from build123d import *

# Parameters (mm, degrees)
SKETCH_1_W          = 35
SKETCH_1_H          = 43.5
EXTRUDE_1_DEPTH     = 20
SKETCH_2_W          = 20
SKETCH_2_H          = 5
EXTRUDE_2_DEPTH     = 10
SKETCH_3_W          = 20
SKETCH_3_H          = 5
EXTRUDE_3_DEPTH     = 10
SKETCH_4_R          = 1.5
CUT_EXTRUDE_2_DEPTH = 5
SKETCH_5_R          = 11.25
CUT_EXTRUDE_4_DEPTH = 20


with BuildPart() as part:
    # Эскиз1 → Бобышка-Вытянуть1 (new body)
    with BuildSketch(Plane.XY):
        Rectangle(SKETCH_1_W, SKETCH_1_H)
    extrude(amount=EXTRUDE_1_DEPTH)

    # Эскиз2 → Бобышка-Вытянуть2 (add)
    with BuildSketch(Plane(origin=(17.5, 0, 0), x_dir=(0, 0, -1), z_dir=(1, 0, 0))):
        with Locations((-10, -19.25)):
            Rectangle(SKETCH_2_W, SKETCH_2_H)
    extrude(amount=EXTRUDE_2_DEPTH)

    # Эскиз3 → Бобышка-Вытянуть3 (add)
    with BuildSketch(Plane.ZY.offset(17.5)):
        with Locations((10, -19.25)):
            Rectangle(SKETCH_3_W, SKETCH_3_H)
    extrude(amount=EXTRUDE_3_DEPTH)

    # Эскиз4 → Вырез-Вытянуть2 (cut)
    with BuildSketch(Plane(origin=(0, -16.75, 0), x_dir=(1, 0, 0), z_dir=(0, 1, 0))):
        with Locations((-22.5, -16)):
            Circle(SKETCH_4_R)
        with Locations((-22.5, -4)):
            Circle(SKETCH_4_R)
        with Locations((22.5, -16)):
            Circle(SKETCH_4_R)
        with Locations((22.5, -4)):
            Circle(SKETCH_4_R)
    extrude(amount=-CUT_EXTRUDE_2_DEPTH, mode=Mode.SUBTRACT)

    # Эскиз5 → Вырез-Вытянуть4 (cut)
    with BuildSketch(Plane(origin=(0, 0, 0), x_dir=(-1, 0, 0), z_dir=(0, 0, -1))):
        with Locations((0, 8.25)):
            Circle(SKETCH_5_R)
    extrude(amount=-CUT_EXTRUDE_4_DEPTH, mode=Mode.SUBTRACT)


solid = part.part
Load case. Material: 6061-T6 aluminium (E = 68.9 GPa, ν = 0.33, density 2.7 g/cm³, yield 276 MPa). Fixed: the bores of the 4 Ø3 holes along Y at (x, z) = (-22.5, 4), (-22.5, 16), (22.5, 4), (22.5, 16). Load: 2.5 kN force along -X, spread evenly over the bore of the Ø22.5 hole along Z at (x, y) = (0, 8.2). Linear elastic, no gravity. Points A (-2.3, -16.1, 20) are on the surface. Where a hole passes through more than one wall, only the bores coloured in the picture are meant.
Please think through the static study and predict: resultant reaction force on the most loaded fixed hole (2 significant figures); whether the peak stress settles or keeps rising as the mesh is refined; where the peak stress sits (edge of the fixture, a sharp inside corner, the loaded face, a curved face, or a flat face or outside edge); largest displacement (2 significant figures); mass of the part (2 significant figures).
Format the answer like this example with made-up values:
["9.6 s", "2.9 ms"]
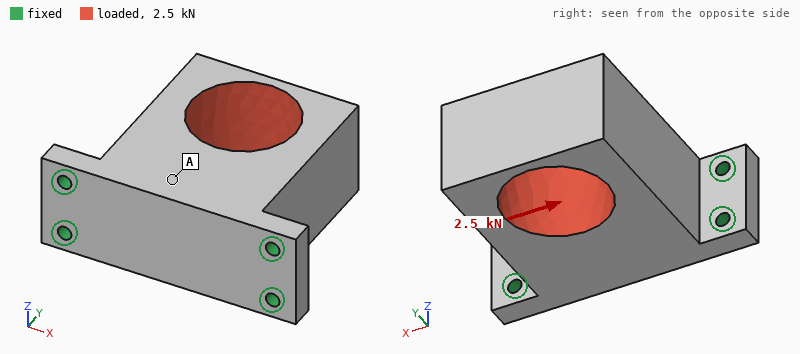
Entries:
["1.1 kN", "keeps rising", "edge of the fixture", "55 µm", "66 g"]
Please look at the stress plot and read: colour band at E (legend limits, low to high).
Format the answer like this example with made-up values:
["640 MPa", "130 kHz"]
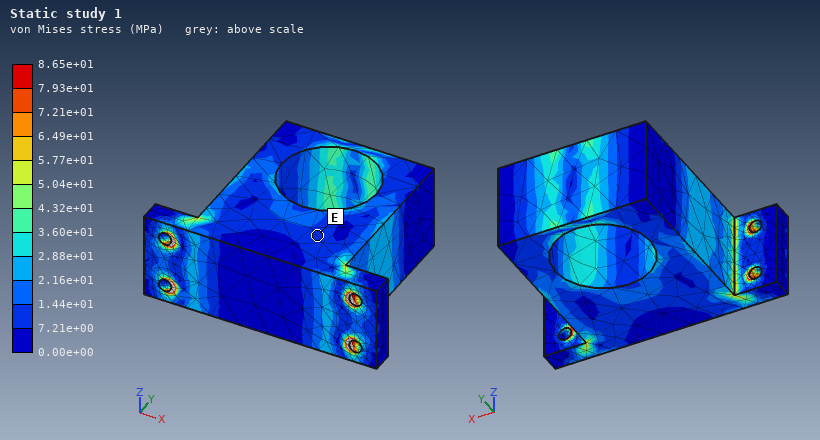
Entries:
["7.21e+00 to 1.44e+01 MPa"]
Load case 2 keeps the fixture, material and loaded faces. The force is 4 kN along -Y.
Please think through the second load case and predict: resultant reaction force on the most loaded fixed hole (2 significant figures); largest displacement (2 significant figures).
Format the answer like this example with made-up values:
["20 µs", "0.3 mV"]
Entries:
["1.1 kN", "25 µm"]
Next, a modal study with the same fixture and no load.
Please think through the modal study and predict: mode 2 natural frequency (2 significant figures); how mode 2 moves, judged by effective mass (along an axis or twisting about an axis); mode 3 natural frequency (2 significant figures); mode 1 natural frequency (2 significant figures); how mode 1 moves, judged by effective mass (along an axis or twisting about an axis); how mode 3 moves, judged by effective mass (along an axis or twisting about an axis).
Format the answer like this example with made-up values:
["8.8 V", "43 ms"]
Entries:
["7100 Hz", "along X", "11 kHz", "3500 Hz", "along Z", "twisting about Y"]
